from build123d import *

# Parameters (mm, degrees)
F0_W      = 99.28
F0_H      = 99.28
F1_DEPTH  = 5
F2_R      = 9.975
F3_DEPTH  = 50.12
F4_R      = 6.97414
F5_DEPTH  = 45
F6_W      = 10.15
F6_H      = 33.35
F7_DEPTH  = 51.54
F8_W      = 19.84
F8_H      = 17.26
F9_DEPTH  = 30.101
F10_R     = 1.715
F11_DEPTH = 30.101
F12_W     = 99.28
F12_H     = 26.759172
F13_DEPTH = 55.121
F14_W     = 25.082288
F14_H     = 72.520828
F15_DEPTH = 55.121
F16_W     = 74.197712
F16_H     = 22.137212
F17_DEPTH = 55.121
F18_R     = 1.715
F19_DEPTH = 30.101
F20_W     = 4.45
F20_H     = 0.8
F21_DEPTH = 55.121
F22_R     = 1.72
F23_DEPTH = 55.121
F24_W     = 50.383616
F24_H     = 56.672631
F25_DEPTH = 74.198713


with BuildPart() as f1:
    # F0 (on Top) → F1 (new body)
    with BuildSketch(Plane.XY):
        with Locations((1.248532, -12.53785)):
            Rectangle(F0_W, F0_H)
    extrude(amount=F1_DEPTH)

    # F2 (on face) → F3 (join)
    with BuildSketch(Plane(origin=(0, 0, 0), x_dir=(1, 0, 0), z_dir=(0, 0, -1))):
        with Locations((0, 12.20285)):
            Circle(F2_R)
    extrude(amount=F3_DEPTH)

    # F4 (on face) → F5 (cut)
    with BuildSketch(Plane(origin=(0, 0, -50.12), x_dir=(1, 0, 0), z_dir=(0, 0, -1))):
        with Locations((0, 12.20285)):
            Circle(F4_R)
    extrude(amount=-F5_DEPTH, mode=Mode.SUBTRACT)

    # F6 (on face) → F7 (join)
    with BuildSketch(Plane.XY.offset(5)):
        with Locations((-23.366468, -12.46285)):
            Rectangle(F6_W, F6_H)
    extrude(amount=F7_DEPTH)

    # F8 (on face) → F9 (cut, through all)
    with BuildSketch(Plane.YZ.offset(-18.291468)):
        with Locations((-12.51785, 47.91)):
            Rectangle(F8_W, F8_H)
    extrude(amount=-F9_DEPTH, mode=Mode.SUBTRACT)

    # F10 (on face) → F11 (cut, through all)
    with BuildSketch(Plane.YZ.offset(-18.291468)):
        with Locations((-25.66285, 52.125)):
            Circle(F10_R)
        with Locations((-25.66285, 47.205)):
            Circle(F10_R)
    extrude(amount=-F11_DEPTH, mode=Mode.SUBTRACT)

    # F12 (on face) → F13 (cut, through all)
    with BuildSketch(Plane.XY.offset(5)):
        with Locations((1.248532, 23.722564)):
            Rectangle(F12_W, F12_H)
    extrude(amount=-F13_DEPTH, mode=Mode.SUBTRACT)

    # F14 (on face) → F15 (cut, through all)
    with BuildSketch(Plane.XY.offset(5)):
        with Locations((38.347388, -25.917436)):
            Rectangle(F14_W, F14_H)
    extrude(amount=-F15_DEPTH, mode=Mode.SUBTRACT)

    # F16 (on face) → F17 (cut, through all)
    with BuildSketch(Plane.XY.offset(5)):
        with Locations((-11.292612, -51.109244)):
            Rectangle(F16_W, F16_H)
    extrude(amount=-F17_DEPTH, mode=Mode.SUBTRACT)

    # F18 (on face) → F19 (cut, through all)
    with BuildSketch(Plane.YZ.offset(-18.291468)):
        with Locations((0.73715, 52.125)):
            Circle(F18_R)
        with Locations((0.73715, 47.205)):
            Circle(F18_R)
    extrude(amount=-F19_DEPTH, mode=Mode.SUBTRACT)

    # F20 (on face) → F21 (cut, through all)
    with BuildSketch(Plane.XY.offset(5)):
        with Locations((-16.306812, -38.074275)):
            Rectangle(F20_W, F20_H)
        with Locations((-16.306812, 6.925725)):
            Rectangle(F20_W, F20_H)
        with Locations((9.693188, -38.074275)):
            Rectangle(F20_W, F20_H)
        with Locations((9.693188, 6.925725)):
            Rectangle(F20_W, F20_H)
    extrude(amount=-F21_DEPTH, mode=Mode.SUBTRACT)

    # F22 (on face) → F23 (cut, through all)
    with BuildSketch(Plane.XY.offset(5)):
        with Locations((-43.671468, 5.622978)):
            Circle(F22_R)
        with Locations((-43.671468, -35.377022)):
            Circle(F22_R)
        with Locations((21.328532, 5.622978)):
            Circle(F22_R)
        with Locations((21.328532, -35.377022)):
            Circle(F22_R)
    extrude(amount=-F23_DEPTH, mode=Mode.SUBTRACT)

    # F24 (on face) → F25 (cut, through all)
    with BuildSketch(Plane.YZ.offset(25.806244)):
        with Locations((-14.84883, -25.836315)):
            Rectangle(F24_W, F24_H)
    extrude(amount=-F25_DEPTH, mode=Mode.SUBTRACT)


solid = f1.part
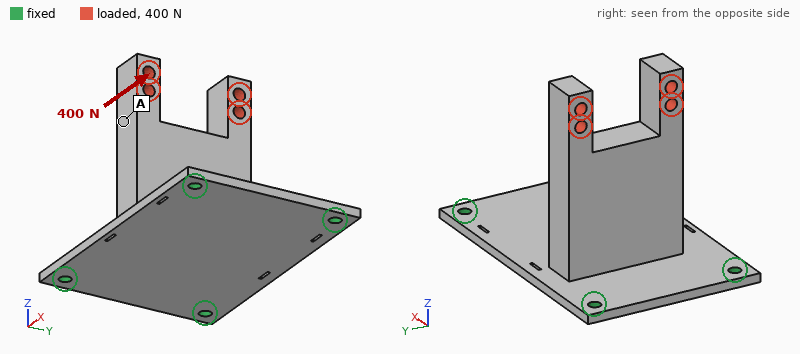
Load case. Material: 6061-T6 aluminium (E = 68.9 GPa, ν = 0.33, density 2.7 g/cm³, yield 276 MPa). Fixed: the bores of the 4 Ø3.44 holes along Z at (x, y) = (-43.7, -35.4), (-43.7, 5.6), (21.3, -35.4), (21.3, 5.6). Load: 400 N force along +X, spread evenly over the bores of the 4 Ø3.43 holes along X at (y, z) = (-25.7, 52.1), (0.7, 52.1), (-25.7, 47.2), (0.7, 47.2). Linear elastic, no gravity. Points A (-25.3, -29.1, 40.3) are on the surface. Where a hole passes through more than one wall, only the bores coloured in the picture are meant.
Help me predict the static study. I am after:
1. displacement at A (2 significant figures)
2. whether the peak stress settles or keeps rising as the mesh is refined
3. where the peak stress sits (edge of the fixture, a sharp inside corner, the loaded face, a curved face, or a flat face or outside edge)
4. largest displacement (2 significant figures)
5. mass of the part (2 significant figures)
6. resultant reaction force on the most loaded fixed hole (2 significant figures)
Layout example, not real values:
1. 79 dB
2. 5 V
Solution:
1. 0.58 mm
2. keeps rising
3. edge of the fixture
4. 0.88 mm
5. 62 g
6. 220 N
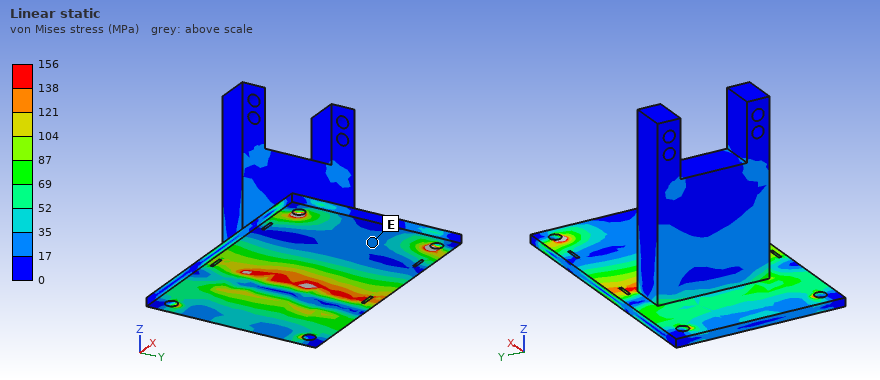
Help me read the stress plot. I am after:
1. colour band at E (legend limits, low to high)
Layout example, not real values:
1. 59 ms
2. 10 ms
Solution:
1. 17 to 35 MPa
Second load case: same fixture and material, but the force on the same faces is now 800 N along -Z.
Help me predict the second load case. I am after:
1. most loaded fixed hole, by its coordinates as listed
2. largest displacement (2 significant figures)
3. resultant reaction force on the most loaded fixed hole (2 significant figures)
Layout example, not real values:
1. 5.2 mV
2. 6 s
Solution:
1. (-43.7, 5.6)
2. 0.37 mm
3. 340 N
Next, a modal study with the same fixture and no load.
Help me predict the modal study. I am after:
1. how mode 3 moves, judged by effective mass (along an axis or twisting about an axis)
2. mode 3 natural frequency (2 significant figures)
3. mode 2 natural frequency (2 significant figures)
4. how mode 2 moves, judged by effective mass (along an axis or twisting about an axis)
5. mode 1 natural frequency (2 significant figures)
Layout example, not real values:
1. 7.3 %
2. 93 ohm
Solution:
1. along Z
2. 2200 Hz
3. 1400 Hz
4. along Y
5. 990 Hz
